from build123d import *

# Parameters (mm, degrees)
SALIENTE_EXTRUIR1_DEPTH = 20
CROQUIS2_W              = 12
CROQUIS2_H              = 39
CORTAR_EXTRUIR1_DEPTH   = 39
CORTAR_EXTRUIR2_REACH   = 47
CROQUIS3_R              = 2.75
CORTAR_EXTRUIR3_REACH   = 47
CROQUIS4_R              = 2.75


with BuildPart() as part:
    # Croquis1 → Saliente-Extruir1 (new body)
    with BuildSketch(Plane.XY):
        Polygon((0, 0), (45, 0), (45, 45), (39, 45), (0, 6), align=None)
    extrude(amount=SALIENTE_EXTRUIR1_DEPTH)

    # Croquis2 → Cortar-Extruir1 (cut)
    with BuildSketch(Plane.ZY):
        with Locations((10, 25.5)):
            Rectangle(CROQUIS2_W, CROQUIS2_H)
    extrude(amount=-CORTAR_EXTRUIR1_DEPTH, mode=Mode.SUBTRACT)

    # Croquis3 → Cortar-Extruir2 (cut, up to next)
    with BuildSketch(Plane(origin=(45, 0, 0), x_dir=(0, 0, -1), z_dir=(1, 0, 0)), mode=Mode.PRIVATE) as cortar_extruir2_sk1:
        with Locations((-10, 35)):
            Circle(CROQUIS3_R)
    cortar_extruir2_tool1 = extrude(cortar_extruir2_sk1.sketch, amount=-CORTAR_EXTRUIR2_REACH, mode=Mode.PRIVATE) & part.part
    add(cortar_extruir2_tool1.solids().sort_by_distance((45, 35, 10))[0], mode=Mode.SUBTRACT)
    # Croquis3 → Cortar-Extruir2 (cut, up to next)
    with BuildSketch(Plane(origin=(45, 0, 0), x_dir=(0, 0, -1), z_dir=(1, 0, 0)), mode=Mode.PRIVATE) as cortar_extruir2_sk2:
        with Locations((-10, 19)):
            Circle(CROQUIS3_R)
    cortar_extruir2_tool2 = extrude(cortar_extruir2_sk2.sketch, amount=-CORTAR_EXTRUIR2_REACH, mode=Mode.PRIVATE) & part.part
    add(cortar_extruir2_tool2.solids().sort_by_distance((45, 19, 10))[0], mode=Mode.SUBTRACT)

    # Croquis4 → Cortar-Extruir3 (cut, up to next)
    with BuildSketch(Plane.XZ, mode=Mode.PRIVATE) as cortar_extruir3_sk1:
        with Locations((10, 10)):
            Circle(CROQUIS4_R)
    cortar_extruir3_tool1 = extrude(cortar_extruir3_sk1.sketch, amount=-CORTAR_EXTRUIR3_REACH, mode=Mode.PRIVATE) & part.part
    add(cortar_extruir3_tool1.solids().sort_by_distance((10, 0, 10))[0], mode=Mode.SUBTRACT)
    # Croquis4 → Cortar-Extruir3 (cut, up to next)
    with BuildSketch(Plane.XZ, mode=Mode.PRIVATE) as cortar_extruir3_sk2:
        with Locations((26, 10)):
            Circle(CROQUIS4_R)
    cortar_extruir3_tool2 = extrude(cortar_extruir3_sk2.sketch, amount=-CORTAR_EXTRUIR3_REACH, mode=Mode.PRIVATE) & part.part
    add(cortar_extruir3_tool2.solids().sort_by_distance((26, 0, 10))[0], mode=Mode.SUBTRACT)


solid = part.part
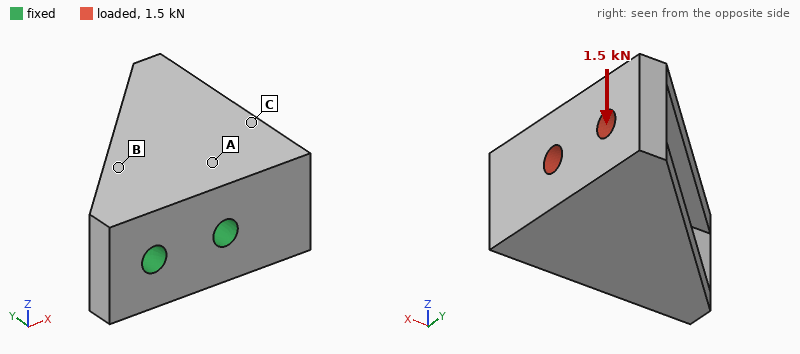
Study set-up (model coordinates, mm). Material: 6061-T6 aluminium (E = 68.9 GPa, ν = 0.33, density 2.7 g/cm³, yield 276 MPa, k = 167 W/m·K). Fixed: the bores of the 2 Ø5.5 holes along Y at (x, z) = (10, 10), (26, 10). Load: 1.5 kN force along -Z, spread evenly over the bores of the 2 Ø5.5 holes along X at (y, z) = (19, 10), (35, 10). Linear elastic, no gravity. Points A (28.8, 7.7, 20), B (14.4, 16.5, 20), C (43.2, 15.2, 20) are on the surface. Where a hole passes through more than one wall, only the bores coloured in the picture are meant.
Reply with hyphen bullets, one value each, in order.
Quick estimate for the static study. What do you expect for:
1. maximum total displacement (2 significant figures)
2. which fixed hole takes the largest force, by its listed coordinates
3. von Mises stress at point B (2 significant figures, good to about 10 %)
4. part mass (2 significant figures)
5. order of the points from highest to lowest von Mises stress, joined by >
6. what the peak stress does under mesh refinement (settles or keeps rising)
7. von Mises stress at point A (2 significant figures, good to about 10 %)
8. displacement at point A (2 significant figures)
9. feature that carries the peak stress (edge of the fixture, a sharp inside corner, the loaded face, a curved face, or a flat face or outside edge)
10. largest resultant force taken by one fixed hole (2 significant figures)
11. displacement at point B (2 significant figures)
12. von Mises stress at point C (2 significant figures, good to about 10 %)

- 0.23 mm
- (26, 10)
- 38 MPa
- 42 g
- A > B > C
- keeps rising
- 65 MPa
- 0.036 mm
- edge of the fixture
- 2.3 kN
- 0.044 mm
- 17 MPa
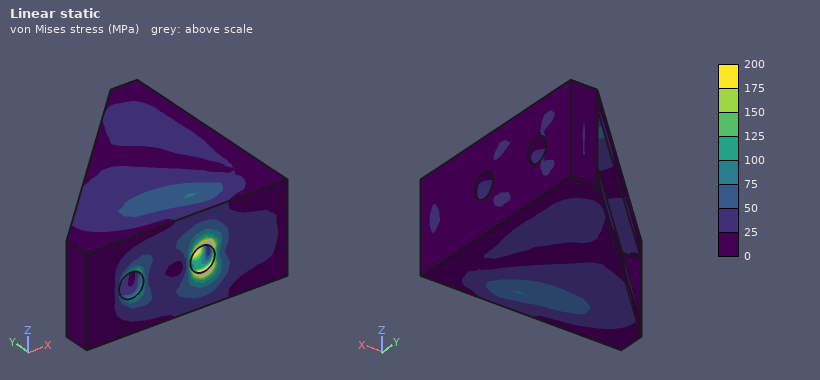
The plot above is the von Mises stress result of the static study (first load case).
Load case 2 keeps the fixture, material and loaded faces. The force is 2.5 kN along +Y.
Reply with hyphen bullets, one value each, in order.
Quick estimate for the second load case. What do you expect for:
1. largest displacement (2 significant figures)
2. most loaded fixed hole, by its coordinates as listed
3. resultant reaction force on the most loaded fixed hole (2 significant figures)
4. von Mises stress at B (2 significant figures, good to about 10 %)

- 76 µm
- (26, 10)
- 3.9 kN
- 23 MPa
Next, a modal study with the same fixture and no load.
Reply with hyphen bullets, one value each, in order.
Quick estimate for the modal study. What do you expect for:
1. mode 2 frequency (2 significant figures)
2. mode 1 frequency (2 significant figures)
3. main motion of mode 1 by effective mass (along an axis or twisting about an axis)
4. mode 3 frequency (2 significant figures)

- 6500 Hz
- 3500 Hz
- along Z
- 12 kHz
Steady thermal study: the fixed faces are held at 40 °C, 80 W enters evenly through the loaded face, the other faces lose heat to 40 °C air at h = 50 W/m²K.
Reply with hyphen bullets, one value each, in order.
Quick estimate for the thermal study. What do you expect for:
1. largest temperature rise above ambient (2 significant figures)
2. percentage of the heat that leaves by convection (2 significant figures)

- 64 K
- 12 %
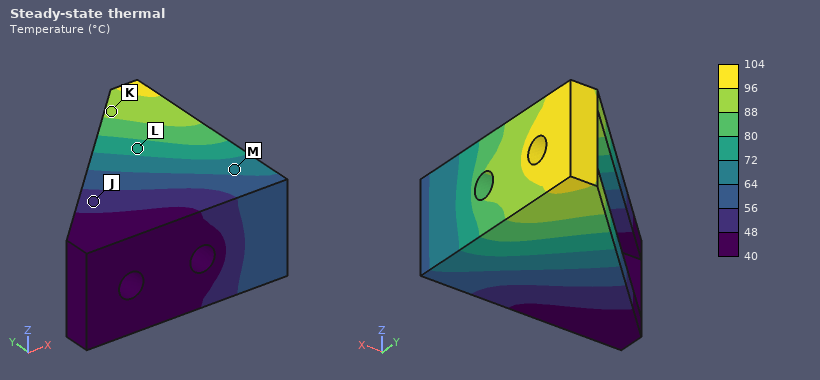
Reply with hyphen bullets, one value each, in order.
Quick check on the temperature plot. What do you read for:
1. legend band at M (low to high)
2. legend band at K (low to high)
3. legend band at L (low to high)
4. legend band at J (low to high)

- 64 to 72 °C
- 88 to 96 °C
- 72 to 80 °C
- 48 to 56 °C
